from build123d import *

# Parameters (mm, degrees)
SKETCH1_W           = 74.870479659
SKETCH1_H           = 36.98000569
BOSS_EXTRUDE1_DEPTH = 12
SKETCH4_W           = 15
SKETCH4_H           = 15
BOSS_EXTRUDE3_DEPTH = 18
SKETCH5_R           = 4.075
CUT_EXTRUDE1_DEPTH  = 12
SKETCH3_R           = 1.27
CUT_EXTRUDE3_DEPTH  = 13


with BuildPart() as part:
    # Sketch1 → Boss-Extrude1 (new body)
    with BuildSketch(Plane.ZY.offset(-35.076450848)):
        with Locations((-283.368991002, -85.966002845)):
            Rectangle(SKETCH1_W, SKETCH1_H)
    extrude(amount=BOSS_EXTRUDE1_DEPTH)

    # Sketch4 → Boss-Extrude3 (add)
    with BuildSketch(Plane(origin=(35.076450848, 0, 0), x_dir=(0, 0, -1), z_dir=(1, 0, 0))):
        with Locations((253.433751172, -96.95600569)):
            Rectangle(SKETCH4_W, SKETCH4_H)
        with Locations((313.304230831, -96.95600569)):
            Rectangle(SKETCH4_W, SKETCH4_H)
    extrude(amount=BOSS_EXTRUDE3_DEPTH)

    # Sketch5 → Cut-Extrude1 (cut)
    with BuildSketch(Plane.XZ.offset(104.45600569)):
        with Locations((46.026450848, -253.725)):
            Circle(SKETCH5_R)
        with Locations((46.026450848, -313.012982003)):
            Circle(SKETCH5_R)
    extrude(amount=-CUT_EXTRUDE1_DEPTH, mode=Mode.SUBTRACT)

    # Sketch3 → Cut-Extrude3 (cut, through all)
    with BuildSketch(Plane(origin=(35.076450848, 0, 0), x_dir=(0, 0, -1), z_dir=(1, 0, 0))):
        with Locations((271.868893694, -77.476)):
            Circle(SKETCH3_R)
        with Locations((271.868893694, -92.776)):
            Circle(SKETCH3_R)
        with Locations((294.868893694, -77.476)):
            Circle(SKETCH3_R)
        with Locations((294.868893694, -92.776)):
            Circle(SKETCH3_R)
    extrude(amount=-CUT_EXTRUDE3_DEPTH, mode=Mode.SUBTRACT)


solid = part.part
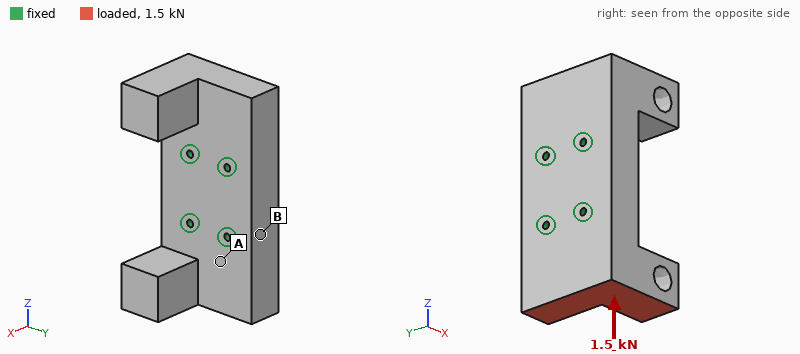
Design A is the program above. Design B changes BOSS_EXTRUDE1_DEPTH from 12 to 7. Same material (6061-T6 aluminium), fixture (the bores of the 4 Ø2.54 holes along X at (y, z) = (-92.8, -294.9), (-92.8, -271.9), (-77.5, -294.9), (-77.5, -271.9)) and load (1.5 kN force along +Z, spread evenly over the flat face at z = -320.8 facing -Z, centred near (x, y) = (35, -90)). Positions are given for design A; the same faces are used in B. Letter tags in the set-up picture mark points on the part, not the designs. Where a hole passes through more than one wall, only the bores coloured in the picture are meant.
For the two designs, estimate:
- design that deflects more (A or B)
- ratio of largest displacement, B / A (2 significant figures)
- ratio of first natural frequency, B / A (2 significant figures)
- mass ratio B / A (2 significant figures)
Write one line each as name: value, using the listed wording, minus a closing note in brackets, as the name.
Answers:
design that deflects more: B
ratio of largest displacement, B / A: 3.6
ratio of first natural frequency, B / A: 0.58
mass ratio B / A: 0.65
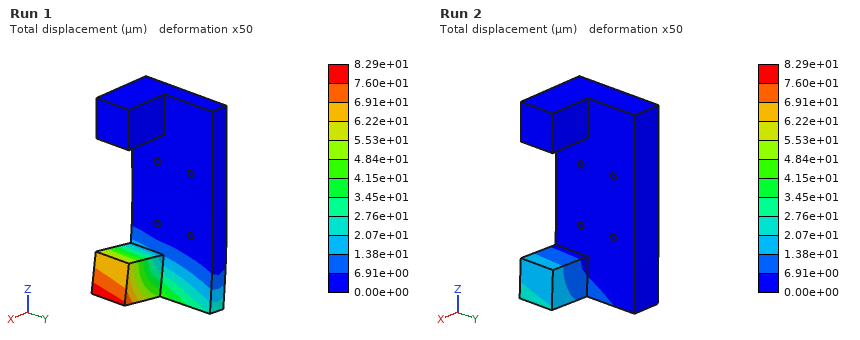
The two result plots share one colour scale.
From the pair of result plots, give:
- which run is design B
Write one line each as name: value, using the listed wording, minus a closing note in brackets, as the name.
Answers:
which run is design B: Run 1
